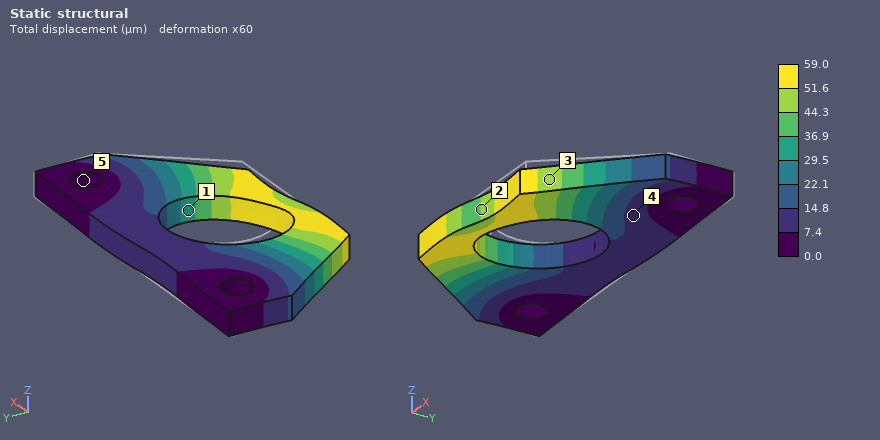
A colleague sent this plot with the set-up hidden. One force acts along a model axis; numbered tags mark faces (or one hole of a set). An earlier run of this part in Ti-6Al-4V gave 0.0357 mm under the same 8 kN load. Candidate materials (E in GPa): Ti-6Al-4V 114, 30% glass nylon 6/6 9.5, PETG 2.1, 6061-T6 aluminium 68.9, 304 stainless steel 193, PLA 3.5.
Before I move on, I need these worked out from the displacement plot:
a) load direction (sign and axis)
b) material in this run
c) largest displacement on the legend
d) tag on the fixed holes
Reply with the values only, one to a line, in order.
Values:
-X
6061-T6 aluminium
59.0 µm
5
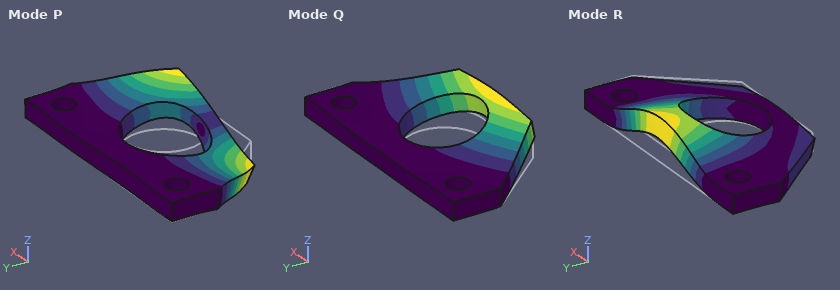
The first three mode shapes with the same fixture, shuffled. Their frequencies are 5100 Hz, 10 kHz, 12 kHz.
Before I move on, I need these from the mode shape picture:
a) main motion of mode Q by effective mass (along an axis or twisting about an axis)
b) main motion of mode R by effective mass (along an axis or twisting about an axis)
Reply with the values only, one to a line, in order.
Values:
along Z
along Z
